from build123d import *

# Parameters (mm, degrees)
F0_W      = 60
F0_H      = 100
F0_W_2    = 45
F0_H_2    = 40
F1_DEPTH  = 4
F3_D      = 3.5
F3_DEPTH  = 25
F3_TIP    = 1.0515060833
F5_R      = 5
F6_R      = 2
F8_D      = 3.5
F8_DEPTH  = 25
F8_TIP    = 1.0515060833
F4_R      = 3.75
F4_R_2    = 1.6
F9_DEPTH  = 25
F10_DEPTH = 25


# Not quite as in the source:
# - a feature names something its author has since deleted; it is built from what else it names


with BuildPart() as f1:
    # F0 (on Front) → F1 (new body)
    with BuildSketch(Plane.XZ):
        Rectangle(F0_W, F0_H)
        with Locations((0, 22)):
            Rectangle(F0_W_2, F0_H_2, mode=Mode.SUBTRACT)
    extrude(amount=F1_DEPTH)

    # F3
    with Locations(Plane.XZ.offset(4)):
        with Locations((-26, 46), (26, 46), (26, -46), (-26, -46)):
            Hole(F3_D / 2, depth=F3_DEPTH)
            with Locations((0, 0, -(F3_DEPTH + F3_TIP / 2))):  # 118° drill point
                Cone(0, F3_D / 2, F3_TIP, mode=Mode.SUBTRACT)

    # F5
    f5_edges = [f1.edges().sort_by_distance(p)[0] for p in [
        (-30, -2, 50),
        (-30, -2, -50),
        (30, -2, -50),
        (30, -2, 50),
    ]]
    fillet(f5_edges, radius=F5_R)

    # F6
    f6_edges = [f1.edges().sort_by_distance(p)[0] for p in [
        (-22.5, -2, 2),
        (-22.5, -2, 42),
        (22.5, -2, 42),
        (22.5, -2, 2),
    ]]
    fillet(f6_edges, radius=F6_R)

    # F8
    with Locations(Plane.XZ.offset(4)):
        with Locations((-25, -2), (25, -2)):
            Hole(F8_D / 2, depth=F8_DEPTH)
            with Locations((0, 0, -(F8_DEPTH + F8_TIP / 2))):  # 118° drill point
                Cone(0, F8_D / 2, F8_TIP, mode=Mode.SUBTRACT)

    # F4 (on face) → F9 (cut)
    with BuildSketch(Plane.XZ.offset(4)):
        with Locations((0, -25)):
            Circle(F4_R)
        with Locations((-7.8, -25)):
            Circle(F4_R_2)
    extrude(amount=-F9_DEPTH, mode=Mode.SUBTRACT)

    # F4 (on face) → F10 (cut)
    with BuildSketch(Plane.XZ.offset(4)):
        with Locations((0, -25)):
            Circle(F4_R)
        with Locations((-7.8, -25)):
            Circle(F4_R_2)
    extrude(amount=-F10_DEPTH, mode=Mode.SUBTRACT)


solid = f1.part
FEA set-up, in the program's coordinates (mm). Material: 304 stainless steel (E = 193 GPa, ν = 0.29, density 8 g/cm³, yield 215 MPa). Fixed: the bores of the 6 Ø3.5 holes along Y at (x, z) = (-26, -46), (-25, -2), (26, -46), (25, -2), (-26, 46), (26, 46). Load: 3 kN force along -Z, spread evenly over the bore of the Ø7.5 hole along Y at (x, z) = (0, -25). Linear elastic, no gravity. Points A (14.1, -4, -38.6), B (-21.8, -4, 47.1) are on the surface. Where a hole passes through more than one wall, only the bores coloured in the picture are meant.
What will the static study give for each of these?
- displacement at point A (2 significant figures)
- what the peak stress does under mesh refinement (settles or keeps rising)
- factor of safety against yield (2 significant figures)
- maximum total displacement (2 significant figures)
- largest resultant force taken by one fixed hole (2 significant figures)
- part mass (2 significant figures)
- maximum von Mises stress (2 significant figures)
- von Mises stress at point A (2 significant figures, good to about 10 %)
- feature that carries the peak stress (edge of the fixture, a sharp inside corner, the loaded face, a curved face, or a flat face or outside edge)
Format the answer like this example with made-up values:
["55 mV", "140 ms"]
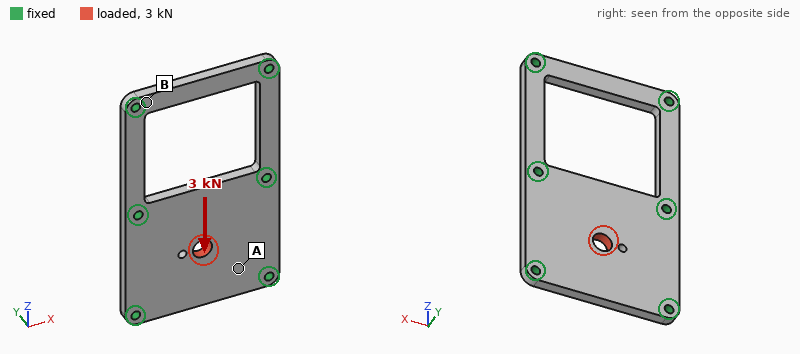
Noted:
["1.9 µm", "settles", "3.6", "4.1 µm", "920 N", "130 g", "59 MPa", "16 MPa", "the loaded face"]
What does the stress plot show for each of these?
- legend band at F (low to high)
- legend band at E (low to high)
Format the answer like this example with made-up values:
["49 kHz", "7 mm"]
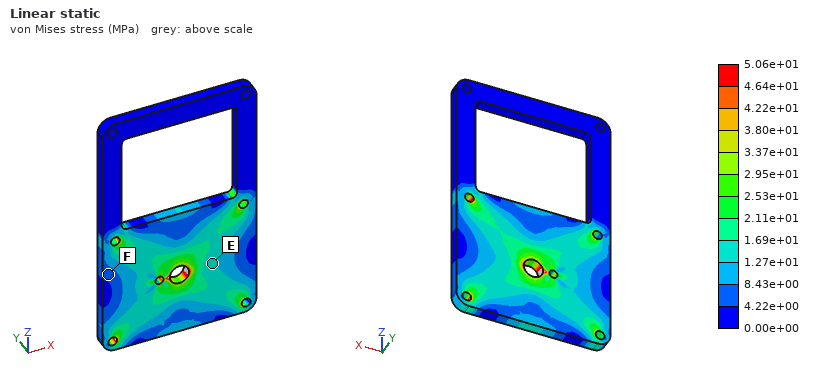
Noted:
["4.22e+00 to 8.43e+00 MPa", "1.27e+01 to 1.69e+01 MPa"]
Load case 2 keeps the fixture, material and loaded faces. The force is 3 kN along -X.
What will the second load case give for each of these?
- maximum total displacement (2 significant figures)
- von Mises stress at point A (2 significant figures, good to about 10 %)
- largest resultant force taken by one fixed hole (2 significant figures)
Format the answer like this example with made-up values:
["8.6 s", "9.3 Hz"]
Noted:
["3.8 µm", "15 MPa", "840 N"]
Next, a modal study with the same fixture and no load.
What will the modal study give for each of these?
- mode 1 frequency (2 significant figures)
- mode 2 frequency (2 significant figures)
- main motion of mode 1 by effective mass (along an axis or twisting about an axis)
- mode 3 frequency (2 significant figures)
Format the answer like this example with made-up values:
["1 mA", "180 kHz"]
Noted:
["5500 Hz", "7800 Hz", "along Y", "8900 Hz"]
